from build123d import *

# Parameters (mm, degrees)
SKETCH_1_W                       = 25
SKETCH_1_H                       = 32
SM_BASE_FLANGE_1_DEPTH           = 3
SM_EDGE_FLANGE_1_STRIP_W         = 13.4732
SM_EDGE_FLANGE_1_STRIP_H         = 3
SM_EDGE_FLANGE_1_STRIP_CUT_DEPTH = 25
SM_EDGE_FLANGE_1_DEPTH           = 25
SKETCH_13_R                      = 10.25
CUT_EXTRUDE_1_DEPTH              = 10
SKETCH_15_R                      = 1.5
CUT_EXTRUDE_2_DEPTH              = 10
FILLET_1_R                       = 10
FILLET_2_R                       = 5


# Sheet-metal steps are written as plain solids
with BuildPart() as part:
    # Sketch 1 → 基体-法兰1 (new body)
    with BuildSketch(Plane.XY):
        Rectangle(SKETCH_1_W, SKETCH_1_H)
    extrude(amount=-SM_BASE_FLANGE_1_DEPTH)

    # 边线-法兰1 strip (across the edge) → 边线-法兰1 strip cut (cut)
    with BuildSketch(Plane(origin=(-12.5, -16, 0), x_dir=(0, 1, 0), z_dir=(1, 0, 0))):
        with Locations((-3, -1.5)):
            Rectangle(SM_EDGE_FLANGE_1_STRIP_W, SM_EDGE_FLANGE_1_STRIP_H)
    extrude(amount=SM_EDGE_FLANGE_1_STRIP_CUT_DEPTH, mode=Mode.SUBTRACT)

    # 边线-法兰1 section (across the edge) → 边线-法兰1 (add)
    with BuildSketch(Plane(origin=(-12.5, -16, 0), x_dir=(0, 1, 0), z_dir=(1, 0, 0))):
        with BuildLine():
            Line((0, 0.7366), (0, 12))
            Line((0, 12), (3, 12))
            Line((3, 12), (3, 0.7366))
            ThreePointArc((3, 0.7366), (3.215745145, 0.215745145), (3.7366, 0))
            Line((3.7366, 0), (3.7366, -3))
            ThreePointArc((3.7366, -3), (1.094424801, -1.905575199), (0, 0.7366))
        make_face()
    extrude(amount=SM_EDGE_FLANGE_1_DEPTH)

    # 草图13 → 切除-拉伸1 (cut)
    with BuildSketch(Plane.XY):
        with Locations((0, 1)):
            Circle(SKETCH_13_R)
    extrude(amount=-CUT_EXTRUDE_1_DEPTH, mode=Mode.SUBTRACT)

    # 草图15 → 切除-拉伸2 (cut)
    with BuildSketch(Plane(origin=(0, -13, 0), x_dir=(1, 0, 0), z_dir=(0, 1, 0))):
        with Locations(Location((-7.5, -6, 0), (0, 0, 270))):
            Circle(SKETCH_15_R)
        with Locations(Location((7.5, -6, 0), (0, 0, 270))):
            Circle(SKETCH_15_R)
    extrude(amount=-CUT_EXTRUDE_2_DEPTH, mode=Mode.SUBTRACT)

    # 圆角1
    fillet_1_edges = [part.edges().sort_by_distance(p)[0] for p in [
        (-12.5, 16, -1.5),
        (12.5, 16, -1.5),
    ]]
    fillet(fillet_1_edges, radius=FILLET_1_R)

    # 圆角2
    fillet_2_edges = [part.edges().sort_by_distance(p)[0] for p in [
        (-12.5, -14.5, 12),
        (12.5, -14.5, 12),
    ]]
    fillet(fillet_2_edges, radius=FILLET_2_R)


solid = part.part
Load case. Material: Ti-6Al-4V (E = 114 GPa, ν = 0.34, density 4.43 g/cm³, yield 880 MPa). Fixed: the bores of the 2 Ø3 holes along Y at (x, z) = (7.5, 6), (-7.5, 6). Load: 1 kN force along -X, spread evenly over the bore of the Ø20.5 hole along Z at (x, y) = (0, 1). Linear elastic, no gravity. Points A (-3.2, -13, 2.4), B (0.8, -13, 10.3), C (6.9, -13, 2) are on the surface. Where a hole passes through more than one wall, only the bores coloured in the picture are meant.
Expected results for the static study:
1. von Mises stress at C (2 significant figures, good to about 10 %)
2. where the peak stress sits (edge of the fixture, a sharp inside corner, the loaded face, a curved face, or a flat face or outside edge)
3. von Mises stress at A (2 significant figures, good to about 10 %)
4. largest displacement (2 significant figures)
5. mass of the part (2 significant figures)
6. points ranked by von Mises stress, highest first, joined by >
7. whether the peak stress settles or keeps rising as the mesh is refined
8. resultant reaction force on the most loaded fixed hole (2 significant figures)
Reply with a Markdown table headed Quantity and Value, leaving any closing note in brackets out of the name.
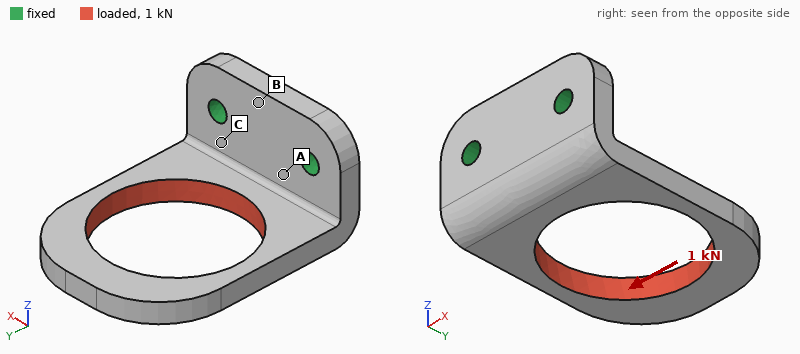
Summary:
| Quantity | Value |
|---|---|
| von Mises stress at C | 150 MPa |
| where the peak stress sits | edge of the fixture |
| von Mises stress at A | 120 MPa |
| largest displacement | 0.23 mm |
| mass of the part | 9.0 g |
| points ranked by von Mises stress, highest first, joined by > | C > A > B |
| whether the peak stress settles or keeps rising as the mesh is refined | keeps rising |
| resultant reaction force on the most loaded fixed hole | 1.1 kN |
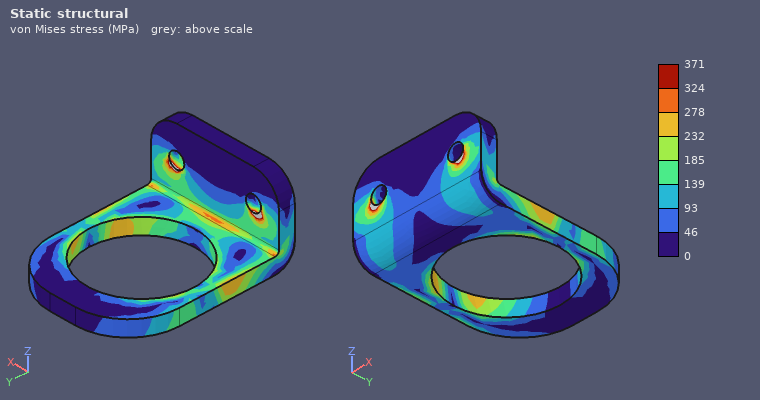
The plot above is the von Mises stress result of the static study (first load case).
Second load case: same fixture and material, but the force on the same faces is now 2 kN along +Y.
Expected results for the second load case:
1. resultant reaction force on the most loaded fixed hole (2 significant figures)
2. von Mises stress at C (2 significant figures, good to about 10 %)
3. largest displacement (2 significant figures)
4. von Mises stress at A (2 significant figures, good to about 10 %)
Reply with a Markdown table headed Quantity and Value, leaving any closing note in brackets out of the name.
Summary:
| Quantity | Value |
|---|---|
| resultant reaction force on the most loaded fixed hole | 1.0 kN |
| von Mises stress at C | 210 MPa |
| largest displacement | 0.27 mm |
| von Mises stress at A | 140 MPa |
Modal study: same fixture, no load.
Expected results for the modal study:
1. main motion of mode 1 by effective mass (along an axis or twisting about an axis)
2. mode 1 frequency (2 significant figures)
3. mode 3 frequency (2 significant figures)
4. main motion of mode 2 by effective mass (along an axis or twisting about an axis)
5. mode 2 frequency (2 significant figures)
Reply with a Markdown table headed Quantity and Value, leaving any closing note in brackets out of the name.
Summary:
| Quantity | Value |
|---|---|
| main motion of mode 1 by effective mass | along Z |
| mode 1 frequency | 2000 Hz |
| mode 3 frequency | 6400 Hz |
| main motion of mode 2 by effective mass | along X |
| mode 2 frequency | 5100 Hz |
